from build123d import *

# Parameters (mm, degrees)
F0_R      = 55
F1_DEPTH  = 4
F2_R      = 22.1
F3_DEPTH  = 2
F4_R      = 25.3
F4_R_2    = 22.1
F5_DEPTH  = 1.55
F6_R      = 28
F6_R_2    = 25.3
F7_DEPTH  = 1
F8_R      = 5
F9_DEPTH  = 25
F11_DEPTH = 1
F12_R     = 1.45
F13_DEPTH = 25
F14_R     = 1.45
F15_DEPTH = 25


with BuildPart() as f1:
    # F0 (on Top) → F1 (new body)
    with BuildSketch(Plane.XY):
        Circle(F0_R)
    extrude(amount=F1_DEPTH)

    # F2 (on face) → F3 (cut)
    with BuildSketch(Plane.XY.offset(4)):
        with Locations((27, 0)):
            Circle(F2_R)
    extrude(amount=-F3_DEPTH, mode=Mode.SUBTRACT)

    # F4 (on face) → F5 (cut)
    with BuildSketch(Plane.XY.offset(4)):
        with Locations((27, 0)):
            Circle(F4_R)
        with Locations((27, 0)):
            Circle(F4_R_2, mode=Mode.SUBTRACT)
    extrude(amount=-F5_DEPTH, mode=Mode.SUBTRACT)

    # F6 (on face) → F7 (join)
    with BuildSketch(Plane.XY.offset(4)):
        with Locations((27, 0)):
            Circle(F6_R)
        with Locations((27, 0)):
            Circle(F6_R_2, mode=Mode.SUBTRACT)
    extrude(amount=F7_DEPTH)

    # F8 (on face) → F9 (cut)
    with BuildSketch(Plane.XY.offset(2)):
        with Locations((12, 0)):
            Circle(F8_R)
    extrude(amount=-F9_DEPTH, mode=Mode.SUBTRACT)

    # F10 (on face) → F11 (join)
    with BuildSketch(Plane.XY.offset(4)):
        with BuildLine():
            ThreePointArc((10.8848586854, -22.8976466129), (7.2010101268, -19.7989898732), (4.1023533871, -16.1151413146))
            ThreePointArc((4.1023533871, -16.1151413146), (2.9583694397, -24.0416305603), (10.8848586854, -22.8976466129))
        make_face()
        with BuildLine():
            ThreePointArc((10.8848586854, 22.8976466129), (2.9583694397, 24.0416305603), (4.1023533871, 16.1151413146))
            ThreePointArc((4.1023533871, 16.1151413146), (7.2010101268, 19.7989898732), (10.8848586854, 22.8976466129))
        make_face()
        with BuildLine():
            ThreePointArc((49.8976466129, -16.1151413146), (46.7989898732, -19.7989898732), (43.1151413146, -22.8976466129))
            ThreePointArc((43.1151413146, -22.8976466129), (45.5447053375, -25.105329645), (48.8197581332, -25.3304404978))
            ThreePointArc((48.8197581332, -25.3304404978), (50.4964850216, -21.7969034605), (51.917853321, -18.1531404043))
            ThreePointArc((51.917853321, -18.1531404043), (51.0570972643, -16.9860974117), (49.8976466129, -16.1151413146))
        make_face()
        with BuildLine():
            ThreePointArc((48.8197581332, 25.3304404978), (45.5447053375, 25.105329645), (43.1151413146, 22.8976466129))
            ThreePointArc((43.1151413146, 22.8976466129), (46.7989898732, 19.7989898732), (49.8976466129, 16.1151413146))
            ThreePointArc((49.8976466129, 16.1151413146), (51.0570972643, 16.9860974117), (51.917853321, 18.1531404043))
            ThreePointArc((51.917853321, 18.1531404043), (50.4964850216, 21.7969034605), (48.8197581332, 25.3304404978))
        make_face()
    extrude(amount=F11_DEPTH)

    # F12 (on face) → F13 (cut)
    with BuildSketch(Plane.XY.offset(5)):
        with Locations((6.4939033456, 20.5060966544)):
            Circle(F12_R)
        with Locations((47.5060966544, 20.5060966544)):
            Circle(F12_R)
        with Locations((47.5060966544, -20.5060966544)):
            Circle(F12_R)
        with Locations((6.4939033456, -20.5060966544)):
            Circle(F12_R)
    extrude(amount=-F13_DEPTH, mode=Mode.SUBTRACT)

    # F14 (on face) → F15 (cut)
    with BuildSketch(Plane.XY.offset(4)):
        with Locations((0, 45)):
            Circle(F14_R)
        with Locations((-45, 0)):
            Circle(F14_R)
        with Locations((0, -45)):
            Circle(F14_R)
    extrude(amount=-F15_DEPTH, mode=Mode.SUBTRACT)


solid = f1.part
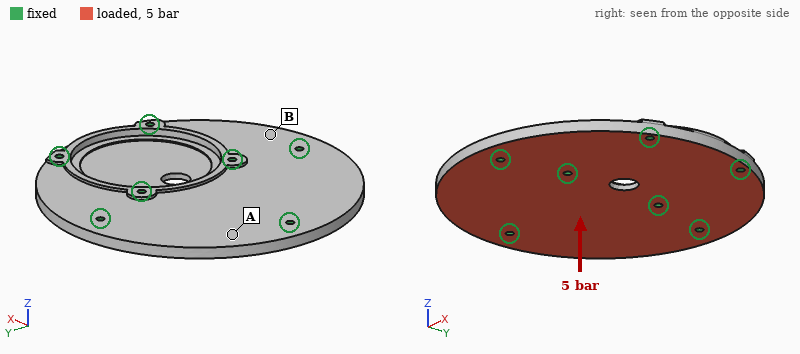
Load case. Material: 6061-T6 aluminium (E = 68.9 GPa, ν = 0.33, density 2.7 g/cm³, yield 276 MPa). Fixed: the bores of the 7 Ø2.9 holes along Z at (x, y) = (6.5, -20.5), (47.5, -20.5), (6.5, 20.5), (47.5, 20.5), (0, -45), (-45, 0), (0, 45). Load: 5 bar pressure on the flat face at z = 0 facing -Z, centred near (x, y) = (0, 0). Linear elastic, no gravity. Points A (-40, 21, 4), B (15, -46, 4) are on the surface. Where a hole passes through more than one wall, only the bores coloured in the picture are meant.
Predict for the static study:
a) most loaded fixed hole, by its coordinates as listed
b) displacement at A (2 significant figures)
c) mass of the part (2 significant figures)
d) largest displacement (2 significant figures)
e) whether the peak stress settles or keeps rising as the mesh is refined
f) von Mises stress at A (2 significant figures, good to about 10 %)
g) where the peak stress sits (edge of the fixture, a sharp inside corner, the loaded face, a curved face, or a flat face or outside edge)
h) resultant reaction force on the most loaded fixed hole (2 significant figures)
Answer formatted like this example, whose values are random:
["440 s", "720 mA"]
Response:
["(-45, 0)", "0.070 mm", "93 g", "0.13 mm", "keeps rising", "24 MPa", "edge of the fixture", "1.0 kN"]
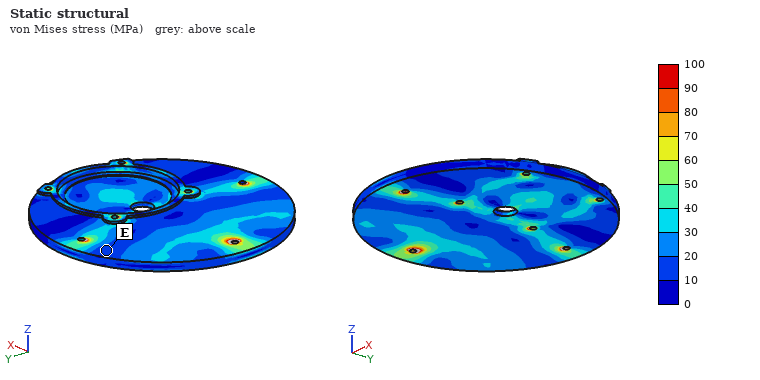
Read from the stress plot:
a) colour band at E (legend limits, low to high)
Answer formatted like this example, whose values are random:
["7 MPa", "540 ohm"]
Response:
["10 to 20 MPa"]
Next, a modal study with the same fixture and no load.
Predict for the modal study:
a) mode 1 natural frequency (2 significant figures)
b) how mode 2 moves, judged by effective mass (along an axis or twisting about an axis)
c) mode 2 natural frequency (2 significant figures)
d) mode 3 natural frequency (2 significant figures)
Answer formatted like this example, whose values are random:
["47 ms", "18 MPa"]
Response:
["3600 Hz", "along Z", "4000 Hz", "6700 Hz"]
